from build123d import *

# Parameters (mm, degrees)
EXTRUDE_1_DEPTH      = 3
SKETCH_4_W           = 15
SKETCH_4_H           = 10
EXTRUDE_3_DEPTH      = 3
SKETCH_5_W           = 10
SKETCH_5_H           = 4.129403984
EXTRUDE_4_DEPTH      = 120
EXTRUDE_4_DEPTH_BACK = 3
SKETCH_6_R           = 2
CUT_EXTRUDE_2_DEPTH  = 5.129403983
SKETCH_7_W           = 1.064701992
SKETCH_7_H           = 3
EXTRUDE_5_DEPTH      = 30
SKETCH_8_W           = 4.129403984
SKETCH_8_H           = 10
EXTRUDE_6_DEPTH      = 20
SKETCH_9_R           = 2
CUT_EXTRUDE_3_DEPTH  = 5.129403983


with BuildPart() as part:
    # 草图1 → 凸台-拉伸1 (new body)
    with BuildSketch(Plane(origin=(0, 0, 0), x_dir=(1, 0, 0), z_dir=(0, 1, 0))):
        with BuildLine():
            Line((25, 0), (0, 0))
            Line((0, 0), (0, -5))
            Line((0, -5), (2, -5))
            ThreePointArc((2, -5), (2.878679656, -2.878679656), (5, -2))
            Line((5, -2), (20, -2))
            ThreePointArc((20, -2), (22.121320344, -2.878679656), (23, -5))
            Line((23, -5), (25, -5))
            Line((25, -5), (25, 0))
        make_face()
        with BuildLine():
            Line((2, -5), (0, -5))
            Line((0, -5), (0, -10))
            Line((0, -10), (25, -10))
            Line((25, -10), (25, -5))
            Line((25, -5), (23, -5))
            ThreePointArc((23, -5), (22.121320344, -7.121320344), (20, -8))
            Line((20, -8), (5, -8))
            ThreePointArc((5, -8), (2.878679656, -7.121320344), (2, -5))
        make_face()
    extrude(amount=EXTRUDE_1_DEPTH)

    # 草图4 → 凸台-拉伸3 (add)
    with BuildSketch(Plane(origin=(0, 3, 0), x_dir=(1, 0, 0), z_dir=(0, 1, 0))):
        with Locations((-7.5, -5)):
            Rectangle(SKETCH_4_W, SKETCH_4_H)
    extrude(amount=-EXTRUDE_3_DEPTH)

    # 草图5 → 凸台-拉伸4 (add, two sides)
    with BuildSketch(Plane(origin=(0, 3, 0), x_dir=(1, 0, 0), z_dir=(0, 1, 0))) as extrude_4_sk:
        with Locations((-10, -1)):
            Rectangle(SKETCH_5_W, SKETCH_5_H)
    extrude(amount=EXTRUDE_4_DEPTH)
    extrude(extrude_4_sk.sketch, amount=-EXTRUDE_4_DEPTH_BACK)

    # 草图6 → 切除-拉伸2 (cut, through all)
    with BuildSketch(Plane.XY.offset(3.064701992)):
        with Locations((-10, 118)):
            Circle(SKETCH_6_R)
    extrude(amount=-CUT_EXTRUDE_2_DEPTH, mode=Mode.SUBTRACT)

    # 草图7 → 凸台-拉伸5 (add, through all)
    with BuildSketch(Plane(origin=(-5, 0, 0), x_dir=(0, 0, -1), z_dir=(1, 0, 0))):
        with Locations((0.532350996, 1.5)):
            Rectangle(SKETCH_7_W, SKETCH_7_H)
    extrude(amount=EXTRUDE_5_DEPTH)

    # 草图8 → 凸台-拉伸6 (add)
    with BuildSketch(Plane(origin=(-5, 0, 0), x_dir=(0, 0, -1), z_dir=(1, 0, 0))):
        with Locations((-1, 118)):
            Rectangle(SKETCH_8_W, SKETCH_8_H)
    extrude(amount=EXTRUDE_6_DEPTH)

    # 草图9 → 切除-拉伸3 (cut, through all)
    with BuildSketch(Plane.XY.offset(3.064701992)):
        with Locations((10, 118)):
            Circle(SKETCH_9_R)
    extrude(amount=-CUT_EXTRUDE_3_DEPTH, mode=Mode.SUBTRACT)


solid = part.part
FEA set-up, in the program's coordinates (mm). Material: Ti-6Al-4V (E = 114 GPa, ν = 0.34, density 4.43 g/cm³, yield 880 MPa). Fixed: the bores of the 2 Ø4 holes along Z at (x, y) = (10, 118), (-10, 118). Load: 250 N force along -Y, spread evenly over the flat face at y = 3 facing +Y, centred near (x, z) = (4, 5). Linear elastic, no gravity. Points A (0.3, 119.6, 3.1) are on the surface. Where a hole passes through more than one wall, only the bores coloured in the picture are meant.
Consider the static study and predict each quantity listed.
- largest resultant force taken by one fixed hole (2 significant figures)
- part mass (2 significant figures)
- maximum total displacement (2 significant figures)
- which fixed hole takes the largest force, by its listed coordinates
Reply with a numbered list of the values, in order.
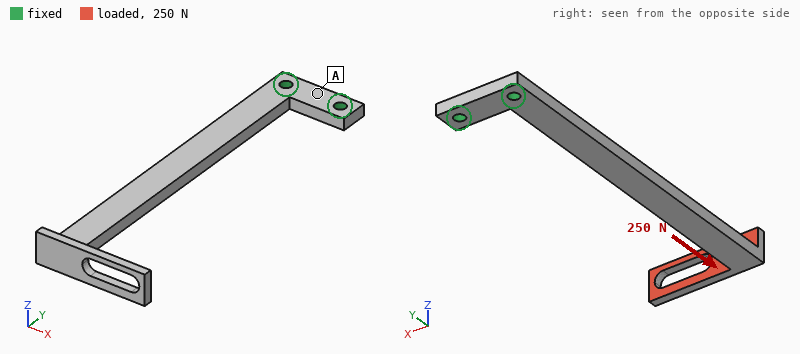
1. 160 N
2. 29 g
3. 1.5 mm
4. (-10, 118)
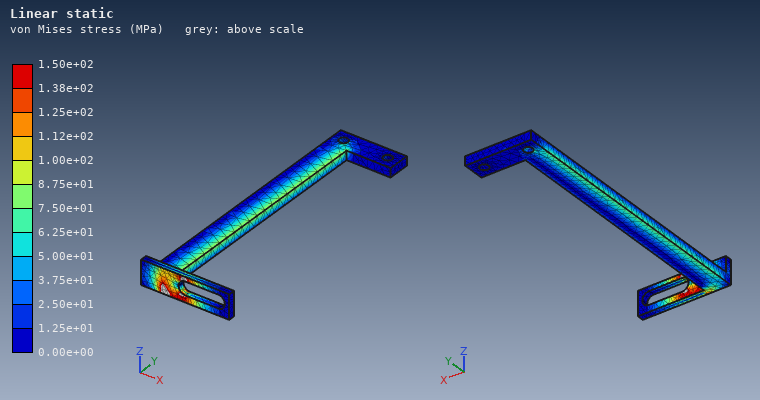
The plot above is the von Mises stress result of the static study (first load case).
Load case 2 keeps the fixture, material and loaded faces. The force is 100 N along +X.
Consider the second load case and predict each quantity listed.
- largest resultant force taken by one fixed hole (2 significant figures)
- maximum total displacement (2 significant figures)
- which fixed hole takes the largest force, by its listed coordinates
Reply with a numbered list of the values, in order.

1. 400 N
2. 1.5 mm
3. (10, 118)
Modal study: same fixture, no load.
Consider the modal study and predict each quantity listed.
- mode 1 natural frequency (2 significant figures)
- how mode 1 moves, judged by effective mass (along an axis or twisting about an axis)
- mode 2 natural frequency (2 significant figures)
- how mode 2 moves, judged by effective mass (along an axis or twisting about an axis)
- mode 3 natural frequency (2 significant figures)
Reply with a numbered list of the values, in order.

1. 190 Hz
2. along Z
3. 450 Hz
4. along X
5. 1100 Hz
